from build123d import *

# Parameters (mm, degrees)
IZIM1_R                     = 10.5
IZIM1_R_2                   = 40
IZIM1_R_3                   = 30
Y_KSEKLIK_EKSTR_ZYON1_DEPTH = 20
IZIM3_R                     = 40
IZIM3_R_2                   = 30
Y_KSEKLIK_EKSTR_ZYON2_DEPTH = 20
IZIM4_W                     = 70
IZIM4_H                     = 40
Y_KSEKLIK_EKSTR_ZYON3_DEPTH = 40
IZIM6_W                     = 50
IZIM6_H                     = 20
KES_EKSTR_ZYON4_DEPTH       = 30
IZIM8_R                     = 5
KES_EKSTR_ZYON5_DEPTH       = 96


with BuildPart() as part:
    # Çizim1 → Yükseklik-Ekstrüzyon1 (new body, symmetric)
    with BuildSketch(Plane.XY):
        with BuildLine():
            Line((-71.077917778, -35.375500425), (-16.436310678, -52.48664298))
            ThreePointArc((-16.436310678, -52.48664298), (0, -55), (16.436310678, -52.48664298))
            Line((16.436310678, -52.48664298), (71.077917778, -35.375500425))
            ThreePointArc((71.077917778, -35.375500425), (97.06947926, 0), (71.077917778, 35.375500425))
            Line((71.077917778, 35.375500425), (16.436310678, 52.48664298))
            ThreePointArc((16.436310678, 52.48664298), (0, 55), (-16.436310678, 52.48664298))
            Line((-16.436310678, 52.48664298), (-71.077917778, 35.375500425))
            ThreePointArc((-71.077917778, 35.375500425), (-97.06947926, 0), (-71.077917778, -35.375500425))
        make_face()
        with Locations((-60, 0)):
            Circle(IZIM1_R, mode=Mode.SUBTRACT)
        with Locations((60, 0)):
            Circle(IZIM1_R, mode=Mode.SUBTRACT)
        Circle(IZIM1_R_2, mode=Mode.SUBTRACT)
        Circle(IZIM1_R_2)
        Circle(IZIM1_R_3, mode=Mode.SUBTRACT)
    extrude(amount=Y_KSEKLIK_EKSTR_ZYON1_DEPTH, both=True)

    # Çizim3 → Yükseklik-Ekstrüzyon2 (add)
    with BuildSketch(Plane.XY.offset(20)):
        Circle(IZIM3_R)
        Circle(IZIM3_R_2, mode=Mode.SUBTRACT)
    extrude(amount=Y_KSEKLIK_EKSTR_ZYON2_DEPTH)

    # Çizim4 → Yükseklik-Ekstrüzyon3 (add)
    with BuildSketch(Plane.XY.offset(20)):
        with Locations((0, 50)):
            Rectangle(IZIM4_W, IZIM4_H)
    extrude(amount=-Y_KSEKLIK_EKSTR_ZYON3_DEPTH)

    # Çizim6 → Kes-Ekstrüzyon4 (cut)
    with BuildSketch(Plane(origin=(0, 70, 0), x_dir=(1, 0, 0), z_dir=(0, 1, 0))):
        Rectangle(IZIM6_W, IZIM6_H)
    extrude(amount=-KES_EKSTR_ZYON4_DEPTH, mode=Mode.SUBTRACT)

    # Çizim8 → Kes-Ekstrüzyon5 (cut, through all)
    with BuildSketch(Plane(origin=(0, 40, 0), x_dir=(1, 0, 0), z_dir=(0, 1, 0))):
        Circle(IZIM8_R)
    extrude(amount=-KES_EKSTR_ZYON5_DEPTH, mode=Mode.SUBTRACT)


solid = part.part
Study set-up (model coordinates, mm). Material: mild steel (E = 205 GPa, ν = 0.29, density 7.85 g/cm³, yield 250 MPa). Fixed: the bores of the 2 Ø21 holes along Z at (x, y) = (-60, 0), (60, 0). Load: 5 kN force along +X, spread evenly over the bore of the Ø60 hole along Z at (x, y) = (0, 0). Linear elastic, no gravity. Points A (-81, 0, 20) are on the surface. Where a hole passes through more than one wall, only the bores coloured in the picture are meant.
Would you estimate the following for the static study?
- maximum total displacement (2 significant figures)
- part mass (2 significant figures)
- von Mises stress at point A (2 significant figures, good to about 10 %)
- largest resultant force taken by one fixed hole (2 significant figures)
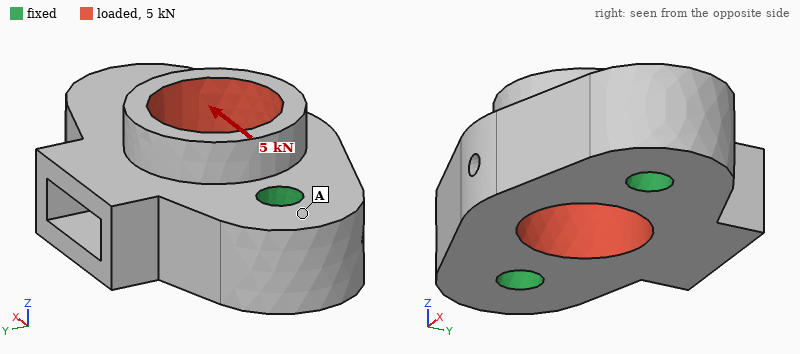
0.67 µm
4.4 kg
0.35 MPa
2.5 kN
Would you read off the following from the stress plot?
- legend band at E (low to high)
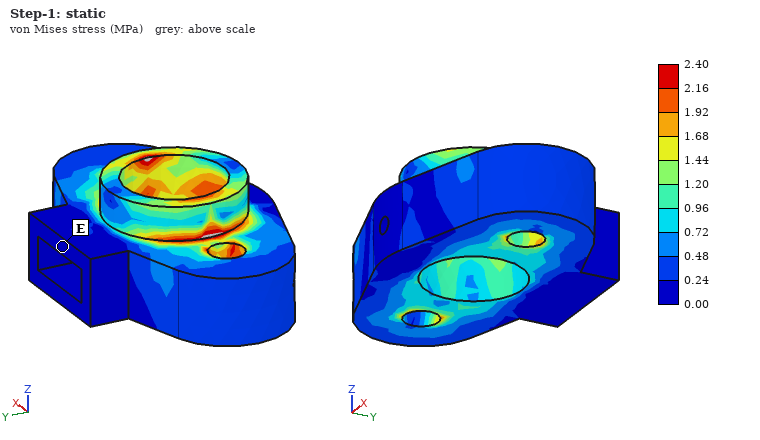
0.00 to 0.24 MPa
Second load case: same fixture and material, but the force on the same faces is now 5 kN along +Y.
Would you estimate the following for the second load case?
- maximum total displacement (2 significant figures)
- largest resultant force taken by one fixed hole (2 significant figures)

1.3 µm
2.5 kN
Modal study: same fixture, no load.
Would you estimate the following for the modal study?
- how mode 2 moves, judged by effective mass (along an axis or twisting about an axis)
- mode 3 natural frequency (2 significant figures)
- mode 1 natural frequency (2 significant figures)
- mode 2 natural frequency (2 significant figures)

along Z
9700 Hz
5800 Hz
7500 Hz
